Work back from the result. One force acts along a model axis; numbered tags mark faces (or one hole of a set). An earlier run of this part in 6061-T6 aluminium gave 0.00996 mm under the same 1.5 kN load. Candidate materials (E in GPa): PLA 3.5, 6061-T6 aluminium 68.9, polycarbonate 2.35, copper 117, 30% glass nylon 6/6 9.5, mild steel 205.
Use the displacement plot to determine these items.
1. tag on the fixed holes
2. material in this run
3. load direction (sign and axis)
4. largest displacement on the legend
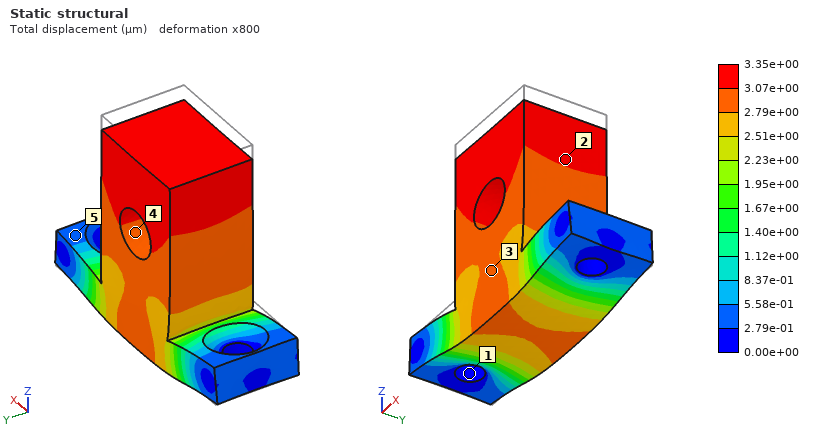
1
mild steel
-Z
3.35e+00 µm
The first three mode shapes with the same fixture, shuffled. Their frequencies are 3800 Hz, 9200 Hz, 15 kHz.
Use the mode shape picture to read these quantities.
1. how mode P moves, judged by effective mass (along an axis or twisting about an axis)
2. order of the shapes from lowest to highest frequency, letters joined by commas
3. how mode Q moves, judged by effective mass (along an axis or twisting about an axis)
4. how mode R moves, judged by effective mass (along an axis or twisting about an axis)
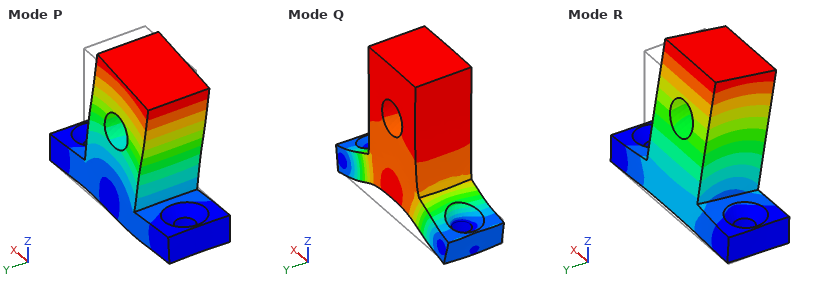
along X
R, P, Q
along Z
along Y
